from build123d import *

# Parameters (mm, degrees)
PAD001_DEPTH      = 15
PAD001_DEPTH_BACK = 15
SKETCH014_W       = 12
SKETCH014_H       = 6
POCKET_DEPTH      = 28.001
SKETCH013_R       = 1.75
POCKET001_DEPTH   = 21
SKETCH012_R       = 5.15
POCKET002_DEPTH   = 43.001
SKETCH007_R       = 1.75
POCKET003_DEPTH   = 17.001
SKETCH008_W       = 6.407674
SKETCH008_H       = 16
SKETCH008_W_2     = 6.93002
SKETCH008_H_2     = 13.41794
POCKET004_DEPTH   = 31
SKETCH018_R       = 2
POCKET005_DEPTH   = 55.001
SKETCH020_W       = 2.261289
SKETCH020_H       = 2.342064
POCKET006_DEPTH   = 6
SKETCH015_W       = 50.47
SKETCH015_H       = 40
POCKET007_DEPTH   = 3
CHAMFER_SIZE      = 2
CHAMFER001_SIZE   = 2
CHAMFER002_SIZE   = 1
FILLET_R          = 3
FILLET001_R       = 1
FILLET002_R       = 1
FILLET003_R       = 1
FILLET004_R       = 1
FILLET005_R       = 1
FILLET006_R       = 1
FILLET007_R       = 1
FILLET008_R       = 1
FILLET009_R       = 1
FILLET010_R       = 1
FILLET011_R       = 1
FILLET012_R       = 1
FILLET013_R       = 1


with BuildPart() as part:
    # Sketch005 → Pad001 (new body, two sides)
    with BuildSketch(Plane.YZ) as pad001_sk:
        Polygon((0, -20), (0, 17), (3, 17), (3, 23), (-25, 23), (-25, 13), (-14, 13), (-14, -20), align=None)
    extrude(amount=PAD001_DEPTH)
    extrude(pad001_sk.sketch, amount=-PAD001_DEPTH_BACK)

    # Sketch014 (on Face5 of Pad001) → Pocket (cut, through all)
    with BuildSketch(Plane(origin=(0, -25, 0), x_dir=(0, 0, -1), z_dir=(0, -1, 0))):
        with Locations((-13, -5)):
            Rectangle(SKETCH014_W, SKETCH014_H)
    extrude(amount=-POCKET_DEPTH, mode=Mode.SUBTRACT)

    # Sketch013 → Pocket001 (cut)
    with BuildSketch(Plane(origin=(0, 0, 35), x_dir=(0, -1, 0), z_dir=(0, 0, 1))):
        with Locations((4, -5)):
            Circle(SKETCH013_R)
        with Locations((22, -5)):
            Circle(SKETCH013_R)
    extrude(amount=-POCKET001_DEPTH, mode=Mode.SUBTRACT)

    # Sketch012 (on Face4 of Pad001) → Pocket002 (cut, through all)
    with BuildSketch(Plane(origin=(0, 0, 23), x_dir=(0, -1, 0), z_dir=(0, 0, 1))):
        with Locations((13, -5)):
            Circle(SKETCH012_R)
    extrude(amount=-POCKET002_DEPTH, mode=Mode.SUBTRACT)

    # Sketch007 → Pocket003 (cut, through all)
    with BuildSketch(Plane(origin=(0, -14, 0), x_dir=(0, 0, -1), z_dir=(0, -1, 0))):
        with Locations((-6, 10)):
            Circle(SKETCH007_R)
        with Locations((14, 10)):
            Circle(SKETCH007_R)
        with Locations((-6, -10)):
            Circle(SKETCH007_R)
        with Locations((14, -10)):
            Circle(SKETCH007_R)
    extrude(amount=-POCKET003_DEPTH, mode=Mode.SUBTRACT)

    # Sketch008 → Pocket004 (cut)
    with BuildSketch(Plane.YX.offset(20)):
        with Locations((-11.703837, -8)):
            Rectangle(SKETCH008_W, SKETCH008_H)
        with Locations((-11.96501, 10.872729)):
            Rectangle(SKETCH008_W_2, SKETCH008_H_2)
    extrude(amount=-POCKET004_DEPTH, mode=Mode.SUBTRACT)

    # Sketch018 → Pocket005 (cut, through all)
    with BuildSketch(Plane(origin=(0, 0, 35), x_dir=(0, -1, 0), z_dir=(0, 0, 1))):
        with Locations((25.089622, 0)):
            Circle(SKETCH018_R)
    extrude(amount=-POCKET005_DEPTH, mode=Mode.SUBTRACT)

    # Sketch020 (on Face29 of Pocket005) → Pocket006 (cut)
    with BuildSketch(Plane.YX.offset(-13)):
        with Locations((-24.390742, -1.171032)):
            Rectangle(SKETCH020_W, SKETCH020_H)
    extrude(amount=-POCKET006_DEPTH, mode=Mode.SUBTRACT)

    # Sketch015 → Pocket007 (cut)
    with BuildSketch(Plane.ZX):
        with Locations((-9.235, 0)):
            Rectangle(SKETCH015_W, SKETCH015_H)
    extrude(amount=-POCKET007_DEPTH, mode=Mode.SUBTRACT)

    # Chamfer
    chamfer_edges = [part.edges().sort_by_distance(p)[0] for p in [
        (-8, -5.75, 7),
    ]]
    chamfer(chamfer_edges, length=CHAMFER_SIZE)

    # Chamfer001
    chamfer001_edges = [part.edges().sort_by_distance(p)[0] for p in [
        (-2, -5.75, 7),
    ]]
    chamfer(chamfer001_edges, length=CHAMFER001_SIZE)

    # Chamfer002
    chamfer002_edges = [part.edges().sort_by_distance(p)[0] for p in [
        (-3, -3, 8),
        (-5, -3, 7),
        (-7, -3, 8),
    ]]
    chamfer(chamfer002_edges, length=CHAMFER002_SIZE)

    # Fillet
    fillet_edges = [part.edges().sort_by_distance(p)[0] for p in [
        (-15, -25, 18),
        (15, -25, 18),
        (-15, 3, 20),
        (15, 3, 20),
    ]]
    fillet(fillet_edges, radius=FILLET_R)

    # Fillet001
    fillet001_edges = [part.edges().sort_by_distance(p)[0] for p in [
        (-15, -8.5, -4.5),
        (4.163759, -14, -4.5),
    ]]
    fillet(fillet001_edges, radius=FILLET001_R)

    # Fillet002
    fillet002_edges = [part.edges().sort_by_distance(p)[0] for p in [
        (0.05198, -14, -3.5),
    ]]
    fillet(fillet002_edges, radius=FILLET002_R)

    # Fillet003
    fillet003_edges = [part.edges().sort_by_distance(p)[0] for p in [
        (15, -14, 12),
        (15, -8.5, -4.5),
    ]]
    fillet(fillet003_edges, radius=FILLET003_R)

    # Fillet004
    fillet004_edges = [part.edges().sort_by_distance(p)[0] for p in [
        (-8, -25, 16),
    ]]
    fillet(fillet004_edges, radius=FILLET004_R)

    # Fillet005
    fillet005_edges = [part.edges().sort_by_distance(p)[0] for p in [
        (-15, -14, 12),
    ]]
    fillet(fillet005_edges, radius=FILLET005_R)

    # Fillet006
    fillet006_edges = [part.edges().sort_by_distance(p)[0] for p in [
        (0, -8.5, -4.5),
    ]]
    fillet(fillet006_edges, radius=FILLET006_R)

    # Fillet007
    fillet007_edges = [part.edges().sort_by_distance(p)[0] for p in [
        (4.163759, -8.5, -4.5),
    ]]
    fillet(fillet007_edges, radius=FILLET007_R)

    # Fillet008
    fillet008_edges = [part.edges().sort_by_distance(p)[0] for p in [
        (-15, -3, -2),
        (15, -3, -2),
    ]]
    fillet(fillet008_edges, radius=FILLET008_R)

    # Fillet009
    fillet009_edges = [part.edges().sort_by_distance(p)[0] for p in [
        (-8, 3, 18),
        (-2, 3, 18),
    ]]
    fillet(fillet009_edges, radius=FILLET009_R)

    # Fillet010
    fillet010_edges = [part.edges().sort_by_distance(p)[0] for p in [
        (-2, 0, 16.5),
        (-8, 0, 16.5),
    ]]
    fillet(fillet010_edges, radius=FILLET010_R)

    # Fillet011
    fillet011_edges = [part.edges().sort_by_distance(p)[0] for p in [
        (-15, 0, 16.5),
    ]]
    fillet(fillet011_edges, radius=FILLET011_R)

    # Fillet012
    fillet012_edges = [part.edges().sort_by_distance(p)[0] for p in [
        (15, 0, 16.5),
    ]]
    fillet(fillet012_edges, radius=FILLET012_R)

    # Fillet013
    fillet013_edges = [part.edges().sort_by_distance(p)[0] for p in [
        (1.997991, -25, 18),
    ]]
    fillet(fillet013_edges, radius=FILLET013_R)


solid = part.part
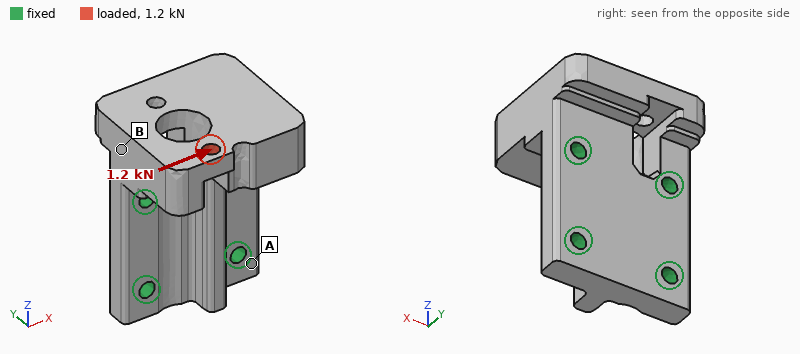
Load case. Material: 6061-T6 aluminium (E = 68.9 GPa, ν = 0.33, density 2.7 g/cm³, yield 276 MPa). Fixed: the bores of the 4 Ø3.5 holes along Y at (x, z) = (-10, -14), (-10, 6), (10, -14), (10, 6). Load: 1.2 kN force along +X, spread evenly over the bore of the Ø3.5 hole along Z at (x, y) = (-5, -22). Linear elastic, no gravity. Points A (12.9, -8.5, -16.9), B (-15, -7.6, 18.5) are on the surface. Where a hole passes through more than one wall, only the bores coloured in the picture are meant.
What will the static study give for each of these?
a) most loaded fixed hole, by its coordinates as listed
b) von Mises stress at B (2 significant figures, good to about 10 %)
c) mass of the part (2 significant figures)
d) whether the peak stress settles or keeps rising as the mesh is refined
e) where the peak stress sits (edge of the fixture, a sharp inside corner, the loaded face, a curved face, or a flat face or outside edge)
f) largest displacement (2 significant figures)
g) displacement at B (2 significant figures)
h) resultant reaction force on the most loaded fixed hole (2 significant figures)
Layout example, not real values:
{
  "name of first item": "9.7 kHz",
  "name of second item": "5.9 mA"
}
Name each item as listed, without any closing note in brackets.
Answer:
{
  "most loaded fixed hole, by its coordinates as listed": "(10, 6)",
  "von Mises stress at B": "17 MPa",
  "mass of the part": "33 g",
  "whether the peak stress settles or keeps rising as the mesh is refined": "keeps rising",
  "where the peak stress sits": "a sharp inside corner",
  "largest displacement": "52 µm",
  "displacement at B": "24 µm",
  "resultant reaction force on the most loaded fixed hole": "1.4 kN"
}
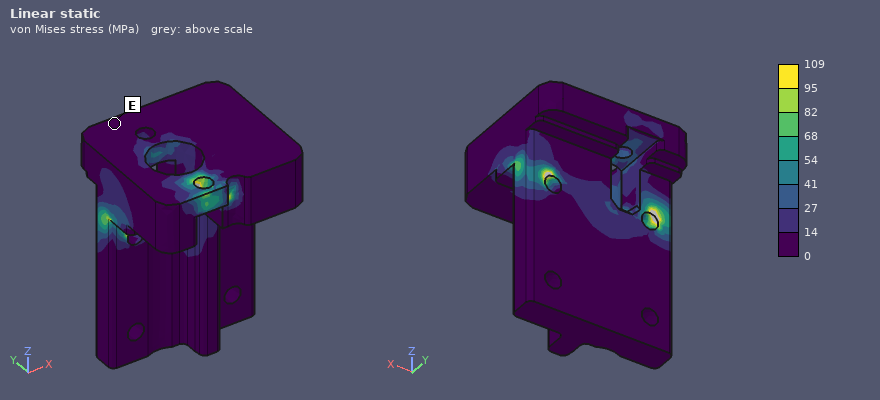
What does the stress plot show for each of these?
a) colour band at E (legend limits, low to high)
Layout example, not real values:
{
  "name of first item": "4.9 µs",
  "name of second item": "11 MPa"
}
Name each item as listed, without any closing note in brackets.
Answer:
{
  "colour band at E": "0 to 14 MPa"
}
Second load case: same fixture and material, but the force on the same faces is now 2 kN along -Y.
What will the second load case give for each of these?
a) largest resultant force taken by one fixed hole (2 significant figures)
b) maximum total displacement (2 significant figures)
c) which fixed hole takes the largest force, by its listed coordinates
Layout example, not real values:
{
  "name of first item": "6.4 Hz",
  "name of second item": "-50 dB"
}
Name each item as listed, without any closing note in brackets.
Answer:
{
  "largest resultant force taken by one fixed hole": "1.5 kN",
  "maximum total displacement": "0.16 mm",
  "which fixed hole takes the largest force, by its listed coordinates": "(-10, 6)"
}
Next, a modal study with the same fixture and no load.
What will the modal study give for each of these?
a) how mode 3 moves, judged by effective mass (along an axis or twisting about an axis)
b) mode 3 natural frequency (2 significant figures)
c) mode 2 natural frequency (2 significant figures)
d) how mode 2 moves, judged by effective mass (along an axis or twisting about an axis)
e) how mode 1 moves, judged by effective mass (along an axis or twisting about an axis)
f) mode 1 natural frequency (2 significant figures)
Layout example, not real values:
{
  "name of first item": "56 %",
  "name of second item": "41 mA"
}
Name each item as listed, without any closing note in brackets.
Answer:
{
  "how mode 3 moves, judged by effective mass": "along X",
  "mode 3 natural frequency": "14 kHz",
  "mode 2 natural frequency": "10 kHz",
  "how mode 2 moves, judged by effective mass": "along X",
  "how mode 1 moves, judged by effective mass": "along Y",
  "mode 1 natural frequency": "6200 Hz"
}
